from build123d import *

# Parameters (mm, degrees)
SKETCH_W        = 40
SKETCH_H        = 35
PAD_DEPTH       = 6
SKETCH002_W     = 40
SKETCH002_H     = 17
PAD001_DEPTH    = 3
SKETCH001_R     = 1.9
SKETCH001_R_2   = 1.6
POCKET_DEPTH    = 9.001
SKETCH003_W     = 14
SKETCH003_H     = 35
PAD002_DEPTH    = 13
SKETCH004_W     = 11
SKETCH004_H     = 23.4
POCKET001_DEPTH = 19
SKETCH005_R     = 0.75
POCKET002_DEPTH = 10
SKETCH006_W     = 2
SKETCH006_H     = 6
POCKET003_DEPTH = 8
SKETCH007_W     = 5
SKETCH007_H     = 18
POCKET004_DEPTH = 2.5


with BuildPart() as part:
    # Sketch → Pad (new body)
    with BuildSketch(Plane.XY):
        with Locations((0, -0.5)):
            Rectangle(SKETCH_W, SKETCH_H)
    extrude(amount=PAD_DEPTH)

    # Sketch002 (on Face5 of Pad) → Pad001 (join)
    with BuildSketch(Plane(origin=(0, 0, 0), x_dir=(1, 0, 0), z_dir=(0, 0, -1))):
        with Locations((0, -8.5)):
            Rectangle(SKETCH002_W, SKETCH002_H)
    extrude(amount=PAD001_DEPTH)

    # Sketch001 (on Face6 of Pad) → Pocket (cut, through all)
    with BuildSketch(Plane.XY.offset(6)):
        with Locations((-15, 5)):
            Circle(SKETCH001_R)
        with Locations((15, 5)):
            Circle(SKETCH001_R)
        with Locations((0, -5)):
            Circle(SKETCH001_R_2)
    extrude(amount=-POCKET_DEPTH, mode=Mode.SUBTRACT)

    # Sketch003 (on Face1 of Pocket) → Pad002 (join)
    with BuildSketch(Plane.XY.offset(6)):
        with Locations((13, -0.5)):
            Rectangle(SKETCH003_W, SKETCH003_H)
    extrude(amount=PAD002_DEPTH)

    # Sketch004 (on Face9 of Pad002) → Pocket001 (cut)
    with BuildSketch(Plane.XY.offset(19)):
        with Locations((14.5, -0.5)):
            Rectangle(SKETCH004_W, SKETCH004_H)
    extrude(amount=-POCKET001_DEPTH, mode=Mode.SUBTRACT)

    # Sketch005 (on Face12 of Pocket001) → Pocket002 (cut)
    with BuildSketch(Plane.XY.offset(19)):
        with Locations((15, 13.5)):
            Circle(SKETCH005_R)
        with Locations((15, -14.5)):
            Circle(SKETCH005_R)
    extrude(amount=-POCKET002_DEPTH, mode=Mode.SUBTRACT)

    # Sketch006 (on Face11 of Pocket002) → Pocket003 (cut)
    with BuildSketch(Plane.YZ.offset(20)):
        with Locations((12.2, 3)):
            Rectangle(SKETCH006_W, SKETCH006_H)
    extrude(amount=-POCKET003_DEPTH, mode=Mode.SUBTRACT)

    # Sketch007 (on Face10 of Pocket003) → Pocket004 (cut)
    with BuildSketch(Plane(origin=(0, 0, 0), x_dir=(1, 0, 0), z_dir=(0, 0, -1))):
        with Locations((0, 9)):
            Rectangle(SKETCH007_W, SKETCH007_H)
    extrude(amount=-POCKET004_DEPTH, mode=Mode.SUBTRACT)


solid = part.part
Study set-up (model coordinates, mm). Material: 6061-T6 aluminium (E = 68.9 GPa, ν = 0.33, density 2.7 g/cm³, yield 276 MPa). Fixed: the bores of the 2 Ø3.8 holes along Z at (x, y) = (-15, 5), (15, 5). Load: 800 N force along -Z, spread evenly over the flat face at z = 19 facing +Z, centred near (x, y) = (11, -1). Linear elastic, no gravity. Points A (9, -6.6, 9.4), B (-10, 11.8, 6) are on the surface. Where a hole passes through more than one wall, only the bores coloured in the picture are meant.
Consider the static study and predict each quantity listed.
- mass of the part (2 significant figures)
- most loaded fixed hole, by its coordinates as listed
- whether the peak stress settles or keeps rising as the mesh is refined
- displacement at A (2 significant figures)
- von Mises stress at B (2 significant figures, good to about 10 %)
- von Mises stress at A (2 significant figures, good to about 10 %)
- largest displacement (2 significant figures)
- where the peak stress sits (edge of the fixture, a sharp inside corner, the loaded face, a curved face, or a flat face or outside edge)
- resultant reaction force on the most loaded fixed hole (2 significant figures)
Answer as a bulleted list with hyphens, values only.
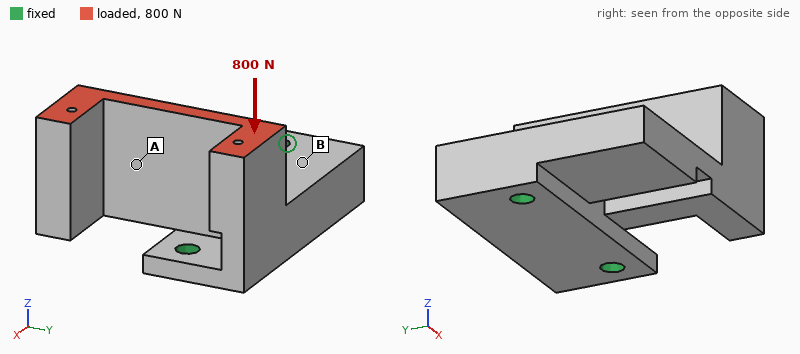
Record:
- 31 g
- (15, 5)
- keeps rising
- 0.038 mm
- 13 MPa
- 29 MPa
- 0.10 mm
- edge of the fixture
- 640 N
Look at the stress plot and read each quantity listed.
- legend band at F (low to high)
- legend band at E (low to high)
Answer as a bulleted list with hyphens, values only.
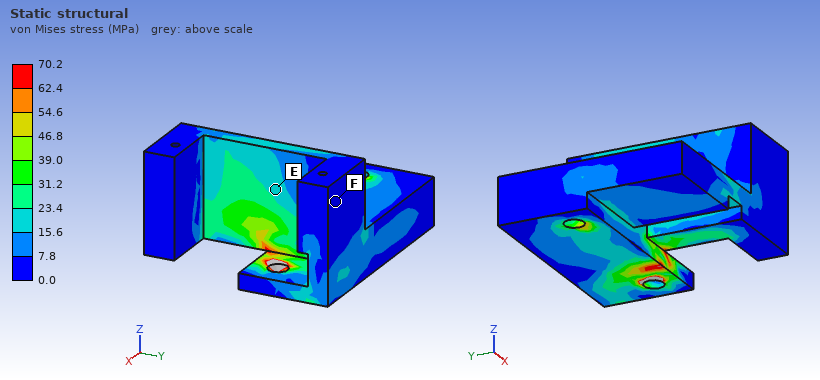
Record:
- 0.0 to 7.8 MPa
- 15.6 to 23.4 MPa
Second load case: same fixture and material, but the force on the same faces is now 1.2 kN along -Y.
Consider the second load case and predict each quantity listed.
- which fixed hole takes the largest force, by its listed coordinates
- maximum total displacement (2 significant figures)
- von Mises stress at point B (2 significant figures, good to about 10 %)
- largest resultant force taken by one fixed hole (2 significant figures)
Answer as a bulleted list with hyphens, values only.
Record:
- (15, 5)
- 0.21 mm
- 61 MPa
- 850 N
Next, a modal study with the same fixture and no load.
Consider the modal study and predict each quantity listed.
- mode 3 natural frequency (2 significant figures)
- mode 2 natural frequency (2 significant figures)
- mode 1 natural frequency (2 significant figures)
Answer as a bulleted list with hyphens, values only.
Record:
- 11 kHz
- 6700 Hz
- 4300 Hz
